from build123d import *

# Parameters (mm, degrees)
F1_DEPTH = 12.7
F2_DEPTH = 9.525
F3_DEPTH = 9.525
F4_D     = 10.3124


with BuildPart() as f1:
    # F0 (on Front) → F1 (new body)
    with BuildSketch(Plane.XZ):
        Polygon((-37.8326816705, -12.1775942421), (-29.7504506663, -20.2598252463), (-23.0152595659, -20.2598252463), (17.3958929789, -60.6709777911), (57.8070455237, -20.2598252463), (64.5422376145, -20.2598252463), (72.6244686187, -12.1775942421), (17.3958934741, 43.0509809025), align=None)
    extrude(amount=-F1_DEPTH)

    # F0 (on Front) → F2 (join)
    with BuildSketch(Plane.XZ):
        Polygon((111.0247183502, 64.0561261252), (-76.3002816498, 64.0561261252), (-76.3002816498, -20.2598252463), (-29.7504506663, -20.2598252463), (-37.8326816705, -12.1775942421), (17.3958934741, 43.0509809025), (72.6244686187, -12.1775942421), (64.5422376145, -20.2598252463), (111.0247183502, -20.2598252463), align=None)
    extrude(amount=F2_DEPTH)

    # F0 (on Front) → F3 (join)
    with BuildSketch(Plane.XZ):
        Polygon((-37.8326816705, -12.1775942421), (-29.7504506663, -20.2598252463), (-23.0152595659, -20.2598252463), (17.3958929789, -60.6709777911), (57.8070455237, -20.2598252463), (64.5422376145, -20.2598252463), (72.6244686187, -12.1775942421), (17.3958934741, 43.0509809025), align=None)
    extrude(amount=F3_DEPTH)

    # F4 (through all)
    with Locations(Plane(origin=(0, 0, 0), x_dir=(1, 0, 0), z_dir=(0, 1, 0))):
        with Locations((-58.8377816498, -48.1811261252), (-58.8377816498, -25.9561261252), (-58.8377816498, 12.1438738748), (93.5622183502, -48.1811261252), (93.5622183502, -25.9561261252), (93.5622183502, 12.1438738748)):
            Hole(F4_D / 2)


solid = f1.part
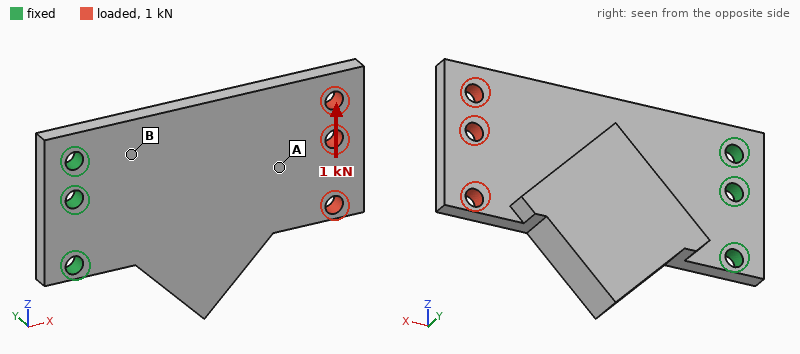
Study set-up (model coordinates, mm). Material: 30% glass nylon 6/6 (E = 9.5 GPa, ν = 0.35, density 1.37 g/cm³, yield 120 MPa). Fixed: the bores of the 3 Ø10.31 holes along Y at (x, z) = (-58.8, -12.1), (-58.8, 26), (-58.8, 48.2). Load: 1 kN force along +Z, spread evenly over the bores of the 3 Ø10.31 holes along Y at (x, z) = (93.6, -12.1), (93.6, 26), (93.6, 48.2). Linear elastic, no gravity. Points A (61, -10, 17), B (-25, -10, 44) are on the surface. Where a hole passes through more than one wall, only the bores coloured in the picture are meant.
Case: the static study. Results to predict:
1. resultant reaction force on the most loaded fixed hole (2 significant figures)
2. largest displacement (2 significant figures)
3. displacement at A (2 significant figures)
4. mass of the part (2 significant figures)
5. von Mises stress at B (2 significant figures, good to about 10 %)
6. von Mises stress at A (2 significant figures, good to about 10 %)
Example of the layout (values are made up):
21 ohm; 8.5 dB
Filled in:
2.4 kN; 0.41 mm; 0.23 mm; 320 g; 5.6 MPa; 2.7 MPa
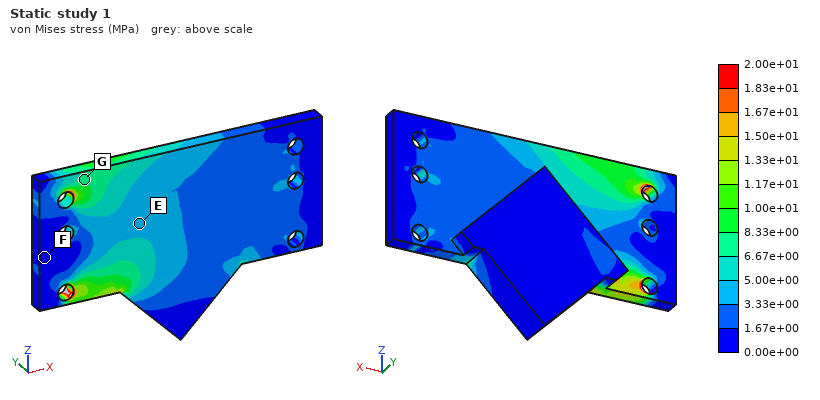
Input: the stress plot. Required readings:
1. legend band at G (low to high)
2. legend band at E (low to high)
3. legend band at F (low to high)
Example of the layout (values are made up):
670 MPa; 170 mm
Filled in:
6.67e+00 to 8.33e+00 MPa; 3.33e+00 to 5.00e+00 MPa; 0.00e+00 to 1.67e+00 MPa
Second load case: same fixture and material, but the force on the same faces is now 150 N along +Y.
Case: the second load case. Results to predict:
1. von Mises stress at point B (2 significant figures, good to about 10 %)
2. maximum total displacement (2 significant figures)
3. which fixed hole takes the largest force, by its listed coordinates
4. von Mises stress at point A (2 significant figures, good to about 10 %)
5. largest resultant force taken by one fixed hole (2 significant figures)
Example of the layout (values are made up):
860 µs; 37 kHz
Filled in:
9.5 MPa; 2.1 mm; (-58.8, 26); 3.0 MPa; 140 N
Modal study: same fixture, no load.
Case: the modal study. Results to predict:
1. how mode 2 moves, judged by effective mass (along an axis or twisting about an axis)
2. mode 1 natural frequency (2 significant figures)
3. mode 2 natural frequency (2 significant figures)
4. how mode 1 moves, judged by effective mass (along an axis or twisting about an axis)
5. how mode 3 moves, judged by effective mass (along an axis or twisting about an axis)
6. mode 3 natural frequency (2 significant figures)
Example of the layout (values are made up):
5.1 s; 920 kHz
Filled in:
twisting about X; 150 Hz; 610 Hz; along Y; along Z; 950 Hz
